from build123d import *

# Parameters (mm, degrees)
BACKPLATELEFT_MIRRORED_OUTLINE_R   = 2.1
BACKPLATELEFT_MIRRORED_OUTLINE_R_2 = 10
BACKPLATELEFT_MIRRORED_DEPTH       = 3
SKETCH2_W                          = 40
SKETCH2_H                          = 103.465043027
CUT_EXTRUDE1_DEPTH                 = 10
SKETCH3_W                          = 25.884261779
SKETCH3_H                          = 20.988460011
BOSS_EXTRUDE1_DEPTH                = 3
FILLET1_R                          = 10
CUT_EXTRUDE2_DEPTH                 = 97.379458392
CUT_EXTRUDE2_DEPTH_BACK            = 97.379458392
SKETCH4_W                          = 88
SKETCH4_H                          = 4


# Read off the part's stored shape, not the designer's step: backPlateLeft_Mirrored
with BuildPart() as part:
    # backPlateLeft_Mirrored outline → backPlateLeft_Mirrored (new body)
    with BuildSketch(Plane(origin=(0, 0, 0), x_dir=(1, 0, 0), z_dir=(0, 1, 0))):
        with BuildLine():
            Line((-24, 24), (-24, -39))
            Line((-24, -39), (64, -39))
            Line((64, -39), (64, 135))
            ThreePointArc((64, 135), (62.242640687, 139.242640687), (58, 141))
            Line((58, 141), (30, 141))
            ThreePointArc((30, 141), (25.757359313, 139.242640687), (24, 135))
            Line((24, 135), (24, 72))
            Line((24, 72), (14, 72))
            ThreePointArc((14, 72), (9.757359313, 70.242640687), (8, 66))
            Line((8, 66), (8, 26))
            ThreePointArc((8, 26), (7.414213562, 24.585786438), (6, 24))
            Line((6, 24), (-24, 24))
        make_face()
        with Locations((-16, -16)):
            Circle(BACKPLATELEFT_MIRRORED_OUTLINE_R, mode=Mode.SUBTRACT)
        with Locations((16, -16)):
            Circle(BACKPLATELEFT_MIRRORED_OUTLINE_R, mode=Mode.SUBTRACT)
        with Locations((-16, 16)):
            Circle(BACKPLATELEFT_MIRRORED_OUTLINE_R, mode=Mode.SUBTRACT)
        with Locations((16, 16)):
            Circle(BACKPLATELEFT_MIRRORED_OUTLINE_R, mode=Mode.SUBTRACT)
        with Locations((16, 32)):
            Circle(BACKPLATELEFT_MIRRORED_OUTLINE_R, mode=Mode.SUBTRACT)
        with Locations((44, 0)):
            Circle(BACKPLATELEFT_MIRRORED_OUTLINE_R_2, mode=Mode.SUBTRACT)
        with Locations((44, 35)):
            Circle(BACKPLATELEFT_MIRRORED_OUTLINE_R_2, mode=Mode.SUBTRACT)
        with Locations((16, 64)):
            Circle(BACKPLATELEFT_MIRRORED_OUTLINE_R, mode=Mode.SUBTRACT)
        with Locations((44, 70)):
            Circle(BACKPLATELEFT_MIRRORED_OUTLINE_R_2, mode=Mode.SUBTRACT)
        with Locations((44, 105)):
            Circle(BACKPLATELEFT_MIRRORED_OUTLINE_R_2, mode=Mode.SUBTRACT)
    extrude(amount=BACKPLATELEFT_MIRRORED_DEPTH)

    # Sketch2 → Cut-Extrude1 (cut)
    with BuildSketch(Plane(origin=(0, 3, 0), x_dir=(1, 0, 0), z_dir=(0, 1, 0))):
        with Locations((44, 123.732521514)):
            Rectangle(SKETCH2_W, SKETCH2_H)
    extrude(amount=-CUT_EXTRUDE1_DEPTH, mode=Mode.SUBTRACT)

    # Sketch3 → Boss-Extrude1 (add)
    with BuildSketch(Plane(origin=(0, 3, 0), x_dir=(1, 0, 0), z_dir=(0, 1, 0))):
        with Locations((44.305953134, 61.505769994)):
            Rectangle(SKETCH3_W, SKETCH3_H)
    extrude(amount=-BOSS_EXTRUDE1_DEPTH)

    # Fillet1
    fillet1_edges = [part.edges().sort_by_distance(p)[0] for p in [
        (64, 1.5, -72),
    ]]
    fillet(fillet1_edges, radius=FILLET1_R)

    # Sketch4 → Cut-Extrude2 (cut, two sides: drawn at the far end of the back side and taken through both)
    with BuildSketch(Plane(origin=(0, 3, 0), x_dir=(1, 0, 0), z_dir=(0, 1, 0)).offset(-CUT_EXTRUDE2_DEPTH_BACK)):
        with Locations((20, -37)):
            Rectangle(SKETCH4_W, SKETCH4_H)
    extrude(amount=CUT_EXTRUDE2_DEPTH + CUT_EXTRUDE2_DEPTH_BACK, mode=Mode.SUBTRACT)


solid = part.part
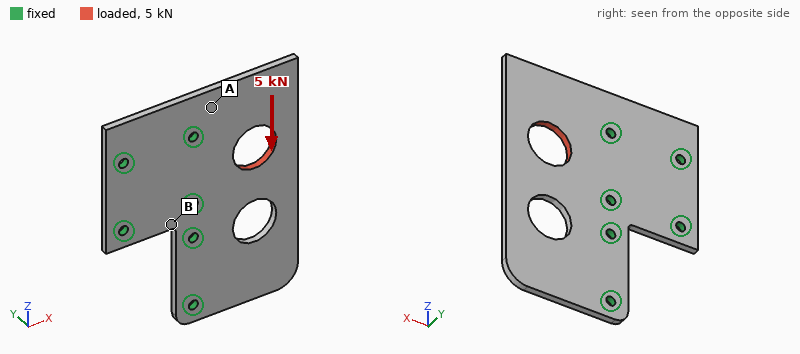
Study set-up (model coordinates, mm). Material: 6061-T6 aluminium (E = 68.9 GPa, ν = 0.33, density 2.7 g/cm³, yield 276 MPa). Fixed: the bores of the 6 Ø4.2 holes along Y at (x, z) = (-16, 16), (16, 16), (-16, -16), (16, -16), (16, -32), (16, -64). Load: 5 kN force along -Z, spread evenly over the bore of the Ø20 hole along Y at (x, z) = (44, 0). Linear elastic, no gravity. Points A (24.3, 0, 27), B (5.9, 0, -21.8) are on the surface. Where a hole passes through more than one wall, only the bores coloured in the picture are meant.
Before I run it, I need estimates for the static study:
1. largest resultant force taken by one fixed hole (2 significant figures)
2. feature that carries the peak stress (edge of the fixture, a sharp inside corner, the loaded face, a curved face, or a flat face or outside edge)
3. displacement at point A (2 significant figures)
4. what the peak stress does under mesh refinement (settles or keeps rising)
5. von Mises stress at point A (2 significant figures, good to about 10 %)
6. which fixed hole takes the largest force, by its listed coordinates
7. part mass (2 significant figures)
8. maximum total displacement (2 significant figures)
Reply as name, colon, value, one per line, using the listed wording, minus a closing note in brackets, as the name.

largest resultant force taken by one fixed hole: 2.4 kN
feature that carries the peak stress: edge of the fixture
displacement at point A: 16 µm
what the peak stress does under mesh refinement: keeps rising
von Mises stress at point A: 23 MPa
which fixed hole takes the largest force, by its listed coordinates: (16, 16)
part mass: 58 g
maximum total displacement: 60 µm
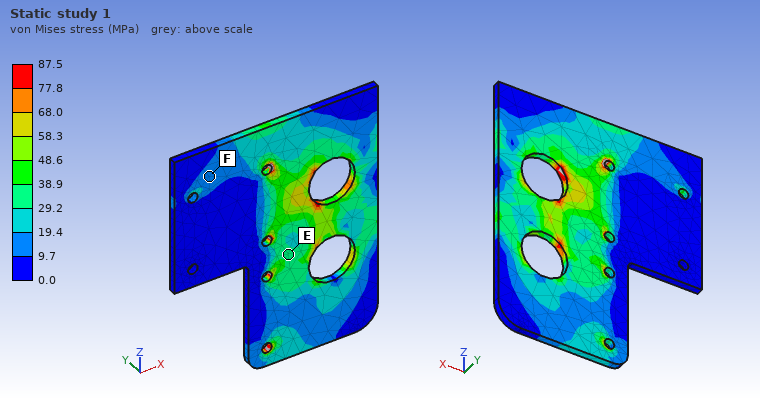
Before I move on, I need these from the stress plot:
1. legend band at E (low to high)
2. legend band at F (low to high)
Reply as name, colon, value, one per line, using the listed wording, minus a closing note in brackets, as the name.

legend band at E: 29.2 to 38.9 MPa
legend band at F: 9.7 to 19.4 MPa
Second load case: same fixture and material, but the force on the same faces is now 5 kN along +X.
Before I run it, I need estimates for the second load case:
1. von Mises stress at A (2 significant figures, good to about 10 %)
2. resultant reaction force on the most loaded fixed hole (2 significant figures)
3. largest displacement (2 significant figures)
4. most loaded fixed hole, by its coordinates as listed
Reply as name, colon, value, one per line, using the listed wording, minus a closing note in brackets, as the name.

von Mises stress at A: 15 MPa
resultant reaction force on the most loaded fixed hole: 2.2 kN
largest displacement: 33 µm
most loaded fixed hole, by its coordinates as listed: (16, 16)
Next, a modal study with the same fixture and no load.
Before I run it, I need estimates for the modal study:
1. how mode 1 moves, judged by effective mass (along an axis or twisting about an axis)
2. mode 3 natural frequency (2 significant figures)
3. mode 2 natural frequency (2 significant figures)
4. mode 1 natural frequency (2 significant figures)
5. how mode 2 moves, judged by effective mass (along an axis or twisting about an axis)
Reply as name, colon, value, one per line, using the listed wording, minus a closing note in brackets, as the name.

how mode 1 moves, judged by effective mass: along Y
mode 3 natural frequency: 2600 Hz
mode 2 natural frequency: 1500 Hz
mode 1 natural frequency: 1100 Hz
how mode 2 moves, judged by effective mass: twisting about X
